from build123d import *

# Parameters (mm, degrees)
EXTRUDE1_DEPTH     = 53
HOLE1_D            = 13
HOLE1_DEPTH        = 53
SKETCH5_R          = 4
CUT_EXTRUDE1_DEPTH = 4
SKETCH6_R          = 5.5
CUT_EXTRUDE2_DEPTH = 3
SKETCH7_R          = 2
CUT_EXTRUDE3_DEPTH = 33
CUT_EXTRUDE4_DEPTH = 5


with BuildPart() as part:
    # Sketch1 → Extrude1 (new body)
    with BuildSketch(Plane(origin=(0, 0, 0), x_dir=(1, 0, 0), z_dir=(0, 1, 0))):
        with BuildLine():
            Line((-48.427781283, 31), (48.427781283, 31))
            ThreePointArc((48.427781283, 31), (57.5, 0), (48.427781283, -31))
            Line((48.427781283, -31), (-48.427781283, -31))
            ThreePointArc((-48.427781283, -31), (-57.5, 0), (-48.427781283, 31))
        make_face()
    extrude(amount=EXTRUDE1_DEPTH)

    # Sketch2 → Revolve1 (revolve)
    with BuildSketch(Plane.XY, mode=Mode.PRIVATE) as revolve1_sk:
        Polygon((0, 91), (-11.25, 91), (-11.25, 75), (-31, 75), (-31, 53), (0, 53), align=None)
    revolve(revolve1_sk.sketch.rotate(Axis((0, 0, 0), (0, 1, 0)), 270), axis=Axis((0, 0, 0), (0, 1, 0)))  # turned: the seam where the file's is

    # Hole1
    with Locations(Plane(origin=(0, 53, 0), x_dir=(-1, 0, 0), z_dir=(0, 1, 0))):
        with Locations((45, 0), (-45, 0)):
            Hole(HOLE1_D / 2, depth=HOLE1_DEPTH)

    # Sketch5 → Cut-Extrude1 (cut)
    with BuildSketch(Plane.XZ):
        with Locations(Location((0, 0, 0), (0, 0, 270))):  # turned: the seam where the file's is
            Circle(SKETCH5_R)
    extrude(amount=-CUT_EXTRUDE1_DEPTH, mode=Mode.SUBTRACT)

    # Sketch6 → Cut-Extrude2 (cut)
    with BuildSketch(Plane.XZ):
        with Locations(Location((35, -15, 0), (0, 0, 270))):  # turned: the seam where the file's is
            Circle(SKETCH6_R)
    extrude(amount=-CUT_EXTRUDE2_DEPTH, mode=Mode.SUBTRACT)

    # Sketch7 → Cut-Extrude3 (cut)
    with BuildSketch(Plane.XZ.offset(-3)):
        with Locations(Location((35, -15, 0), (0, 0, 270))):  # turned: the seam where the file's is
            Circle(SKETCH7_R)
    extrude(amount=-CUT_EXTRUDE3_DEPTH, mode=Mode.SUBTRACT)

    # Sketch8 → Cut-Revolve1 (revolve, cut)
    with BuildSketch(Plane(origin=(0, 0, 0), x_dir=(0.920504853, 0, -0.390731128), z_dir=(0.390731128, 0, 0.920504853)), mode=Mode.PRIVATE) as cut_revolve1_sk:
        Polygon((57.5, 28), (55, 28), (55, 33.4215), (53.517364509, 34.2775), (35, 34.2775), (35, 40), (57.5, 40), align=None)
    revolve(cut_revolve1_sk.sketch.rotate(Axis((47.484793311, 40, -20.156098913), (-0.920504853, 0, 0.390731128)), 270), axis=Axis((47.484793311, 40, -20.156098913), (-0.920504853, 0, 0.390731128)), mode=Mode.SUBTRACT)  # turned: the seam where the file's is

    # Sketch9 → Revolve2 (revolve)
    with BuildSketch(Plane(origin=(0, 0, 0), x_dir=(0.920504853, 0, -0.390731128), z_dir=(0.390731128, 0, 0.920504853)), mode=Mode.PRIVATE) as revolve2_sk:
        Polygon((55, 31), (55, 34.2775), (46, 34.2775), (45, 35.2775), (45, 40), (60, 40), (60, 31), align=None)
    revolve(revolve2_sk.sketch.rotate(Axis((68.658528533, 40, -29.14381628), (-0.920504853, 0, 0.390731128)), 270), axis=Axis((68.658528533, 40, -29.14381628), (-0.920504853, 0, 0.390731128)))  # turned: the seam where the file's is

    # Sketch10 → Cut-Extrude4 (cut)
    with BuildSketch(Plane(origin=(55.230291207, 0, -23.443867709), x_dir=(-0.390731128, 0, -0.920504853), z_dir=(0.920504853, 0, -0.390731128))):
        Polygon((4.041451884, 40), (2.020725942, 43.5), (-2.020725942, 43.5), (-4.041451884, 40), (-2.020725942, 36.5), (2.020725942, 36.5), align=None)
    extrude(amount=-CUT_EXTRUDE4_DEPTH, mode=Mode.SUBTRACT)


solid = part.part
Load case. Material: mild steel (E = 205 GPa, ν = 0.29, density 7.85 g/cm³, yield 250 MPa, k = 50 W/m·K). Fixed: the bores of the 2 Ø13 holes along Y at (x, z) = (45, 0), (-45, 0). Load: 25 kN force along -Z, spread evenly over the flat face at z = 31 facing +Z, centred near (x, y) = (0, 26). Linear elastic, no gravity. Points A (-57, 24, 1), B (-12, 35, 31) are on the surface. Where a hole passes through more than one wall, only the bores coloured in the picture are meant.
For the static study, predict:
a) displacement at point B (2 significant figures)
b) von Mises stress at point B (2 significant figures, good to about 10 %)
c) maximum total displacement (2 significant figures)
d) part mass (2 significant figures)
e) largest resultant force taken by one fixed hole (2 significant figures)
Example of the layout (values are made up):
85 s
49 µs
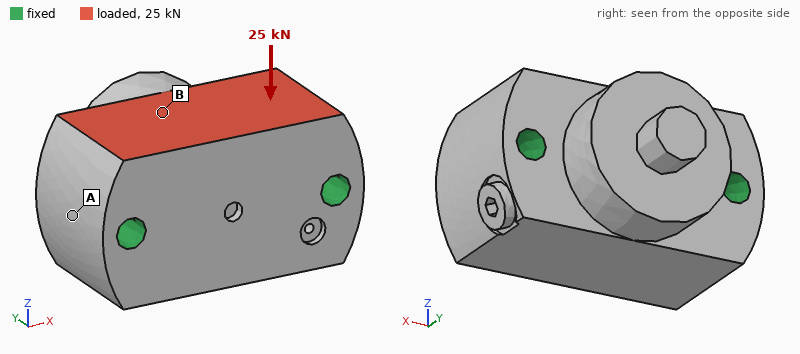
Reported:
1.9 µm
5.1 MPa
2.3 µm
3.3 kg
13 kN
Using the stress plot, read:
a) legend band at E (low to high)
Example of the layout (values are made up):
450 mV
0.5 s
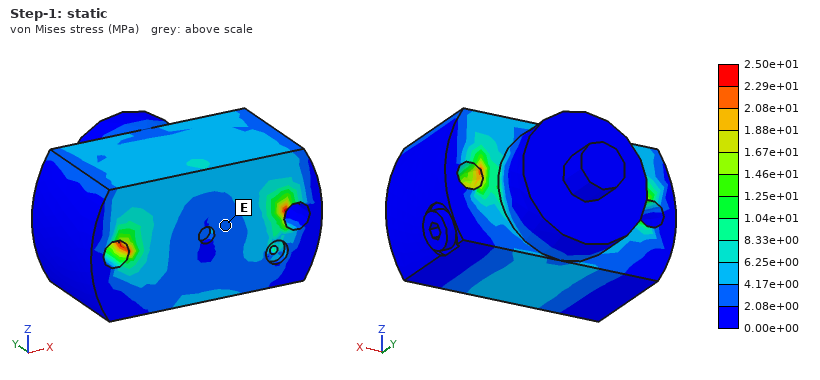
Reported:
2.08e+00 to 4.17e+00 MPa
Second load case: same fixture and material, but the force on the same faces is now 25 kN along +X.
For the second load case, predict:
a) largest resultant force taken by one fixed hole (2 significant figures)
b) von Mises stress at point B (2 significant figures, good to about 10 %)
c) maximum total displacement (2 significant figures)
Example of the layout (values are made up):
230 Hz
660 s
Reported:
15 kN
8.5 MPa
2.4 µm
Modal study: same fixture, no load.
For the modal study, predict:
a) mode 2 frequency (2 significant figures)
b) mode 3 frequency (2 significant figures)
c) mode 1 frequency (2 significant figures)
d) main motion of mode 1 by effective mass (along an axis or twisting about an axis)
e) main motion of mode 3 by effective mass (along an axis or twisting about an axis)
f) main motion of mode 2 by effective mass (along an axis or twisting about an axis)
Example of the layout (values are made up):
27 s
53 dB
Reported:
12 kHz
13 kHz
8400 Hz
along Z
along Z
along Y
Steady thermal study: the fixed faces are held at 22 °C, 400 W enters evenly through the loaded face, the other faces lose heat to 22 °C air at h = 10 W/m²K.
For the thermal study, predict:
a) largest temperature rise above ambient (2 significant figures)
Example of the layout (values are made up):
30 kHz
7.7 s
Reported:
63 K
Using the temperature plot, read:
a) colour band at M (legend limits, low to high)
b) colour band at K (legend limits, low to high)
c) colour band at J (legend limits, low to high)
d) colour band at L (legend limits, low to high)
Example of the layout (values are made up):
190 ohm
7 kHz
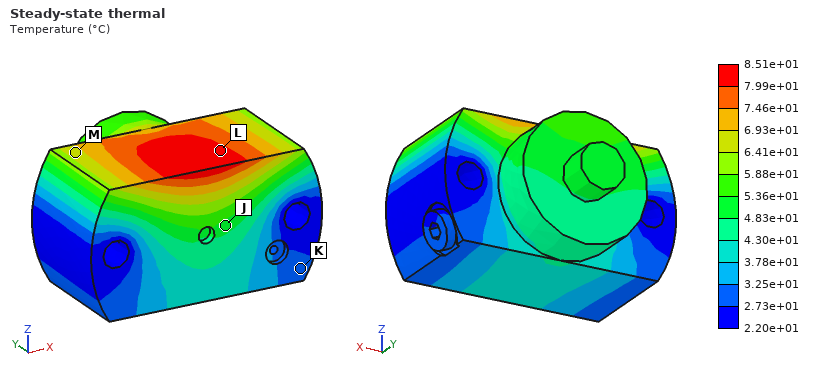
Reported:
6.41e+01 to 6.93e+01 °C
2.73e+01 to 3.25e+01 °C
4.83e+01 to 5.36e+01 °C
7.99e+01 to 8.51e+01 °C
